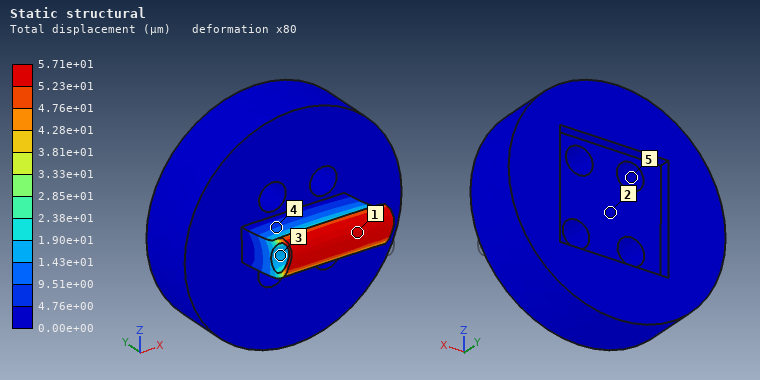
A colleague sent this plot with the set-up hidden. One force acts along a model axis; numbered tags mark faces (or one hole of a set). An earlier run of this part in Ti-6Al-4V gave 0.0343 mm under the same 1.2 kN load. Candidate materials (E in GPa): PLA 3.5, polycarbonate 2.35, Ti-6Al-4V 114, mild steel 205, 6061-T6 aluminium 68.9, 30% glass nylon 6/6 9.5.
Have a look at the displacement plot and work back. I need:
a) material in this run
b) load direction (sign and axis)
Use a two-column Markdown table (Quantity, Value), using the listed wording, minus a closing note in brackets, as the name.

| Quantity | Value |
|---|---|
| material in this run | 6061-T6 aluminium |
| load direction | +Z |
